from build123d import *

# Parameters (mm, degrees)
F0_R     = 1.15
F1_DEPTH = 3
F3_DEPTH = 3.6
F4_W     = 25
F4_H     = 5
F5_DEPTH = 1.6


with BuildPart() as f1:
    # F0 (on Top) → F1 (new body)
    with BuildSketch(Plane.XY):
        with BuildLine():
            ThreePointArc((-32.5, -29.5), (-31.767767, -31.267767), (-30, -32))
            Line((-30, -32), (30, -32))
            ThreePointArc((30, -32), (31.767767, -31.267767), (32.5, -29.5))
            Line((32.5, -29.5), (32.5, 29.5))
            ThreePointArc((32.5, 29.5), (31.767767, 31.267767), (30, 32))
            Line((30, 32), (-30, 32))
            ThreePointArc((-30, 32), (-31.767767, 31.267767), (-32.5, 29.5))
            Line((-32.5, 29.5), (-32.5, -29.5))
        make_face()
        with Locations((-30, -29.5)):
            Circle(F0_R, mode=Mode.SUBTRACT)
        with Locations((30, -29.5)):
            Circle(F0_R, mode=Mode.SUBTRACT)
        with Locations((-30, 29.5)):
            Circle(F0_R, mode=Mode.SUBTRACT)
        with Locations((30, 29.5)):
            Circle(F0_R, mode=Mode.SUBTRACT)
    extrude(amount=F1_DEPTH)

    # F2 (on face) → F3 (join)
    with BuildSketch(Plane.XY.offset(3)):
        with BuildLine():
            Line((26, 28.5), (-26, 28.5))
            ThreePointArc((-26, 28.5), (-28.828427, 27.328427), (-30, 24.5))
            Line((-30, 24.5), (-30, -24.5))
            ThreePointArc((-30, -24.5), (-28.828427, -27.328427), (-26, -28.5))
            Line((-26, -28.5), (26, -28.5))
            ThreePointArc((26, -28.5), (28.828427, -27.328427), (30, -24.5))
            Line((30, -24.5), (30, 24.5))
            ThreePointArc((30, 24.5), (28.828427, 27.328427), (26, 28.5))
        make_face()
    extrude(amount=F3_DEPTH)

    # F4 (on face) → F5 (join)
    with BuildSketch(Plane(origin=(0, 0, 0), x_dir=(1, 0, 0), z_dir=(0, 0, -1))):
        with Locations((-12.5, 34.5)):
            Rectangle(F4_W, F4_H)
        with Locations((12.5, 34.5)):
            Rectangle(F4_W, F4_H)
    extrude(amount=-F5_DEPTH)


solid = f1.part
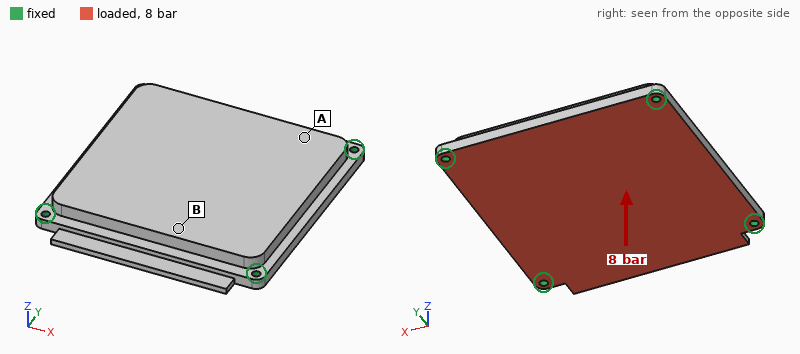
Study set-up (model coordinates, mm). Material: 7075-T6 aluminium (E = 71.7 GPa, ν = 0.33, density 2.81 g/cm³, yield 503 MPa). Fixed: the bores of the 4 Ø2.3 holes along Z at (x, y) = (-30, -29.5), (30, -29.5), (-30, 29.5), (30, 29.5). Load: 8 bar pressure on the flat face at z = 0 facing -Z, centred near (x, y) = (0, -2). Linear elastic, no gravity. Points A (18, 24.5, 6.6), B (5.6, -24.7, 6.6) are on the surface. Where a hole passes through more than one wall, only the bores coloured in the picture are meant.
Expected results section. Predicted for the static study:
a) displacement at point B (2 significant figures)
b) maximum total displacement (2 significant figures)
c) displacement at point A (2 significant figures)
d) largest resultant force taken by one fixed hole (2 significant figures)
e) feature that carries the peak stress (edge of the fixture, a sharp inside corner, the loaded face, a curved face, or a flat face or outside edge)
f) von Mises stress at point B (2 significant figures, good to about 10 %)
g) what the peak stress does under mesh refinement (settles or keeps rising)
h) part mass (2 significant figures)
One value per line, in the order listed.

81 µm
94 µm
48 µm
1.5 kN
edge of the fixture
54 MPa
keeps rising
70 g
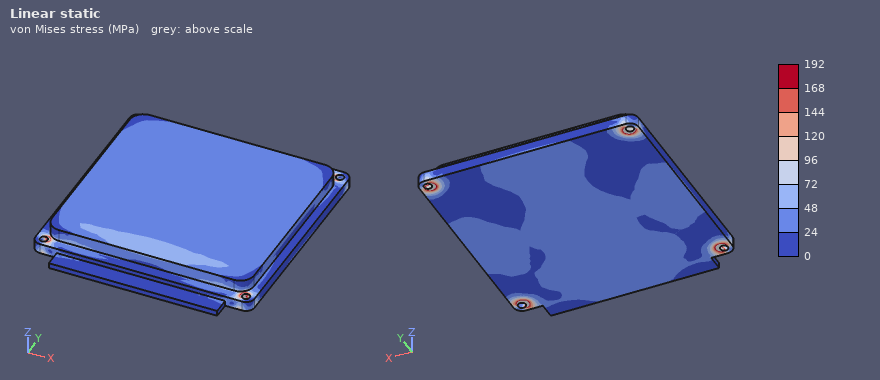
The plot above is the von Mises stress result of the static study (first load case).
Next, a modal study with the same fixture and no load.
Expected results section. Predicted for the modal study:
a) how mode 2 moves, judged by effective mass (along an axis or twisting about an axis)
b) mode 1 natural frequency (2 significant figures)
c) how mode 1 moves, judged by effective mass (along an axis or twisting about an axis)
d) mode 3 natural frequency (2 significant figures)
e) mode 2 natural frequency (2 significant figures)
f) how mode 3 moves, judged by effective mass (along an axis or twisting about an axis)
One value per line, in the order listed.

twisting about X
4000 Hz
along Z
7400 Hz
6900 Hz
twisting about Y
